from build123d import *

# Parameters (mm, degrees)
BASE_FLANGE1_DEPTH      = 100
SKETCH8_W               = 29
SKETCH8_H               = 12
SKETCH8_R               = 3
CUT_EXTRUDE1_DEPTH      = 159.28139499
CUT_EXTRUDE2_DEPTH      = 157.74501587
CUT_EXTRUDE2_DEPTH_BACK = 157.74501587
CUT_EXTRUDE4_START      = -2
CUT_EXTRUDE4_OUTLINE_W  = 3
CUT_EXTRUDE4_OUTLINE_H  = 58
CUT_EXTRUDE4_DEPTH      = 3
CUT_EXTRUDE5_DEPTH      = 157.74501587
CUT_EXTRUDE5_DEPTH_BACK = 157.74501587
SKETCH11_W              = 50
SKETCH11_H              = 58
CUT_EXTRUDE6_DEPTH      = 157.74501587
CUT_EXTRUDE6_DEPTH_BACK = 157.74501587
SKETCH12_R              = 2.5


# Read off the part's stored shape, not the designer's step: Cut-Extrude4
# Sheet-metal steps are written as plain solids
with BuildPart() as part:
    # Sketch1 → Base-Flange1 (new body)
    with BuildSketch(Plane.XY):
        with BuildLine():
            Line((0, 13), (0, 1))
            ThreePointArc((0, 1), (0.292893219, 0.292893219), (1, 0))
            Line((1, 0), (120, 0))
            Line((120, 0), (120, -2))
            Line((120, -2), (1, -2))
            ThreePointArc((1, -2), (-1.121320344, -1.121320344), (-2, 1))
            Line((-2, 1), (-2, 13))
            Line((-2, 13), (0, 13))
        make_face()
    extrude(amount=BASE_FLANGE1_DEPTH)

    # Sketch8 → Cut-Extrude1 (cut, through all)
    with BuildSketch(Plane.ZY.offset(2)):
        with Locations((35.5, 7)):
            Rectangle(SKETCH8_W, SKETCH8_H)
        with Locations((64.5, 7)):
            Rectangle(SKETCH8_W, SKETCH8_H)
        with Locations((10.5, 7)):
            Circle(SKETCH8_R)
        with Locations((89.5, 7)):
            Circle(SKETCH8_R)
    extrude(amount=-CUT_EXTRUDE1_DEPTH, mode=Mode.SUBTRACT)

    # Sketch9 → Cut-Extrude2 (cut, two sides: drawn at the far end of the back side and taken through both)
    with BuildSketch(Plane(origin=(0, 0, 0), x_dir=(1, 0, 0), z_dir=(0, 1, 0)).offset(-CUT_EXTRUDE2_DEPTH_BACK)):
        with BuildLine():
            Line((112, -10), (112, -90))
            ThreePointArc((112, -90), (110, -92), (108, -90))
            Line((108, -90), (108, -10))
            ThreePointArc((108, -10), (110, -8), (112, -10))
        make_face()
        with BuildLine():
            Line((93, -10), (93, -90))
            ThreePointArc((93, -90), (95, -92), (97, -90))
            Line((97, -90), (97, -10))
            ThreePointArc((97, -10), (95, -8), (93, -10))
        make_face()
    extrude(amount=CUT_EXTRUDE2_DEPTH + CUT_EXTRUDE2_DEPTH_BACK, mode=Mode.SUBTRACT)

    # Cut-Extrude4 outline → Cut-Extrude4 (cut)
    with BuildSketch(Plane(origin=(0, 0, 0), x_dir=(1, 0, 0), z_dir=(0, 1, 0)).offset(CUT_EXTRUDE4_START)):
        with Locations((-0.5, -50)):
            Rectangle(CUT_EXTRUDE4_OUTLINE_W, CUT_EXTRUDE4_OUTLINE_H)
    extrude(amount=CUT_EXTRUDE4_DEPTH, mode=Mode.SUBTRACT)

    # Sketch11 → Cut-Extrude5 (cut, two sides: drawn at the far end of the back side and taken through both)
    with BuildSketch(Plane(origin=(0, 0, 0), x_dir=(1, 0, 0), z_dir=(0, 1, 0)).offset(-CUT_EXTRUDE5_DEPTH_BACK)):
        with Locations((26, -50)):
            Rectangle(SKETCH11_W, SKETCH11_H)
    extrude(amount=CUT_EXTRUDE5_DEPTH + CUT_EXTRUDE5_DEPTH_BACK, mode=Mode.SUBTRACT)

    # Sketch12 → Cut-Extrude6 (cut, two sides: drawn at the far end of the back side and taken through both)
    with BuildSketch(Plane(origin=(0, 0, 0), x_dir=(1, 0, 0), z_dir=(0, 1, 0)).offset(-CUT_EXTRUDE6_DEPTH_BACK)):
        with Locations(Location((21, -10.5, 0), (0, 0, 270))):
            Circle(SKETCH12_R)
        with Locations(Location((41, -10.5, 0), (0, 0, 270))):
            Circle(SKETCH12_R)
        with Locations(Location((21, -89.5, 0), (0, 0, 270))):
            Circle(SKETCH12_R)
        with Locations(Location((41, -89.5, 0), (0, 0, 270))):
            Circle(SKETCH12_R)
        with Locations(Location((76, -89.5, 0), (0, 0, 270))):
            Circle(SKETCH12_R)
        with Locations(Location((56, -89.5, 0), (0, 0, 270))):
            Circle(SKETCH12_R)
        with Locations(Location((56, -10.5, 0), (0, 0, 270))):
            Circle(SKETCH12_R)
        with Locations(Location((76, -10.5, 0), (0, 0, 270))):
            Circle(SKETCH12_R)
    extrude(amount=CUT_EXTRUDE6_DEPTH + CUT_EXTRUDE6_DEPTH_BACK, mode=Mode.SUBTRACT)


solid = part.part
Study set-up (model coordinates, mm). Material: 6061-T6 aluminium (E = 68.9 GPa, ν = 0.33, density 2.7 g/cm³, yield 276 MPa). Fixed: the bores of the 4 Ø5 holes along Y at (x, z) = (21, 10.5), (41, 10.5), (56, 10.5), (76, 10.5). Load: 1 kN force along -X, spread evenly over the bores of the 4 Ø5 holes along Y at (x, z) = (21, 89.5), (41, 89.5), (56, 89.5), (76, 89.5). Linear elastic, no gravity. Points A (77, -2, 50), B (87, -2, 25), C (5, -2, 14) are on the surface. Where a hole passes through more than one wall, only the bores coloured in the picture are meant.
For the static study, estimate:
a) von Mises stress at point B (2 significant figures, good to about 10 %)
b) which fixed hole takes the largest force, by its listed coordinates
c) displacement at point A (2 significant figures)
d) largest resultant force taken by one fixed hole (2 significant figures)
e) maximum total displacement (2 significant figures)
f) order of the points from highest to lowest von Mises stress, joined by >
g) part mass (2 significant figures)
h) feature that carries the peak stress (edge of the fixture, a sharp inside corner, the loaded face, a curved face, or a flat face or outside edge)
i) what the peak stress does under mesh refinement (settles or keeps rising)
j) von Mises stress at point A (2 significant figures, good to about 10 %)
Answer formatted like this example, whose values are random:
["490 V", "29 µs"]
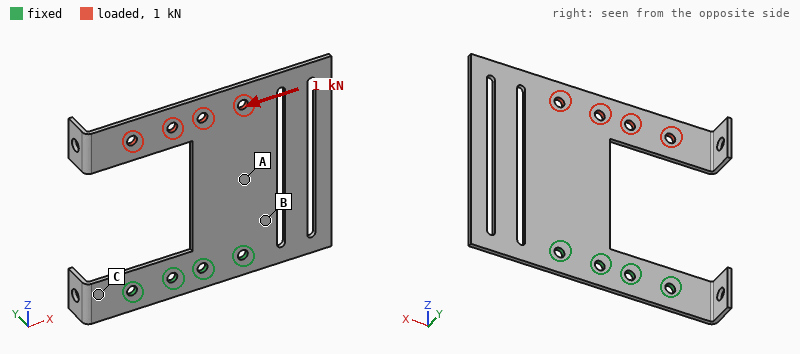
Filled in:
["55 MPa", "(76, 10.5)", "0.11 mm", "3.0 kN", "0.45 mm", "B > A > C", "47 g", "edge of the fixture", "keeps rising", "31 MPa"]
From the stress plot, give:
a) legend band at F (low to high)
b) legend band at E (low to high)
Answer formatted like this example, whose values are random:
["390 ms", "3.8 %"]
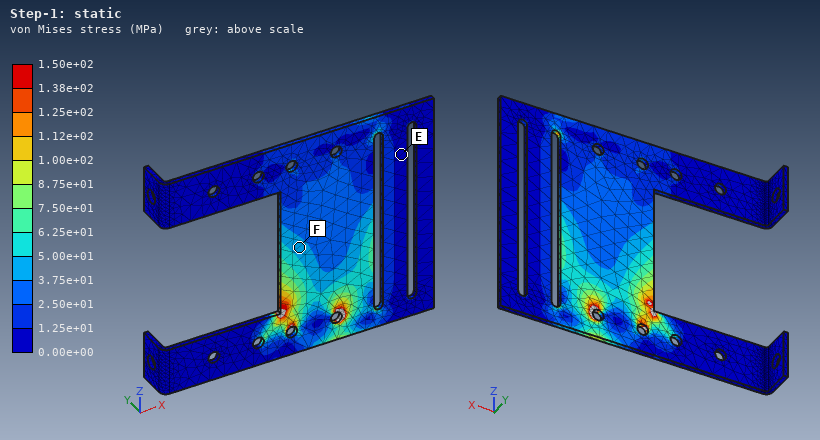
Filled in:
["3.75e+01 to 5.00e+01 MPa", "0.00e+00 to 1.25e+01 MPa"]
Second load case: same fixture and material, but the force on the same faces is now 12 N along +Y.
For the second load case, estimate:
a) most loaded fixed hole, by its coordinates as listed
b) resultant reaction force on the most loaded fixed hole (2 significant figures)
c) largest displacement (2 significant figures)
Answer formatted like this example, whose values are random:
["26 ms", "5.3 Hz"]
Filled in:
["(56, 10.5)", "13 N", "1.6 mm"]
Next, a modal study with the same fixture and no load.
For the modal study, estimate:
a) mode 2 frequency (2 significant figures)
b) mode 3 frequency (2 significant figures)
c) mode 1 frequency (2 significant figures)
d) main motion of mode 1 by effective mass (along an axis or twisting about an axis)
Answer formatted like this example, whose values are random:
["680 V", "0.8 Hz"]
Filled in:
["210 Hz", "510 Hz", "130 Hz", "along Y"]
